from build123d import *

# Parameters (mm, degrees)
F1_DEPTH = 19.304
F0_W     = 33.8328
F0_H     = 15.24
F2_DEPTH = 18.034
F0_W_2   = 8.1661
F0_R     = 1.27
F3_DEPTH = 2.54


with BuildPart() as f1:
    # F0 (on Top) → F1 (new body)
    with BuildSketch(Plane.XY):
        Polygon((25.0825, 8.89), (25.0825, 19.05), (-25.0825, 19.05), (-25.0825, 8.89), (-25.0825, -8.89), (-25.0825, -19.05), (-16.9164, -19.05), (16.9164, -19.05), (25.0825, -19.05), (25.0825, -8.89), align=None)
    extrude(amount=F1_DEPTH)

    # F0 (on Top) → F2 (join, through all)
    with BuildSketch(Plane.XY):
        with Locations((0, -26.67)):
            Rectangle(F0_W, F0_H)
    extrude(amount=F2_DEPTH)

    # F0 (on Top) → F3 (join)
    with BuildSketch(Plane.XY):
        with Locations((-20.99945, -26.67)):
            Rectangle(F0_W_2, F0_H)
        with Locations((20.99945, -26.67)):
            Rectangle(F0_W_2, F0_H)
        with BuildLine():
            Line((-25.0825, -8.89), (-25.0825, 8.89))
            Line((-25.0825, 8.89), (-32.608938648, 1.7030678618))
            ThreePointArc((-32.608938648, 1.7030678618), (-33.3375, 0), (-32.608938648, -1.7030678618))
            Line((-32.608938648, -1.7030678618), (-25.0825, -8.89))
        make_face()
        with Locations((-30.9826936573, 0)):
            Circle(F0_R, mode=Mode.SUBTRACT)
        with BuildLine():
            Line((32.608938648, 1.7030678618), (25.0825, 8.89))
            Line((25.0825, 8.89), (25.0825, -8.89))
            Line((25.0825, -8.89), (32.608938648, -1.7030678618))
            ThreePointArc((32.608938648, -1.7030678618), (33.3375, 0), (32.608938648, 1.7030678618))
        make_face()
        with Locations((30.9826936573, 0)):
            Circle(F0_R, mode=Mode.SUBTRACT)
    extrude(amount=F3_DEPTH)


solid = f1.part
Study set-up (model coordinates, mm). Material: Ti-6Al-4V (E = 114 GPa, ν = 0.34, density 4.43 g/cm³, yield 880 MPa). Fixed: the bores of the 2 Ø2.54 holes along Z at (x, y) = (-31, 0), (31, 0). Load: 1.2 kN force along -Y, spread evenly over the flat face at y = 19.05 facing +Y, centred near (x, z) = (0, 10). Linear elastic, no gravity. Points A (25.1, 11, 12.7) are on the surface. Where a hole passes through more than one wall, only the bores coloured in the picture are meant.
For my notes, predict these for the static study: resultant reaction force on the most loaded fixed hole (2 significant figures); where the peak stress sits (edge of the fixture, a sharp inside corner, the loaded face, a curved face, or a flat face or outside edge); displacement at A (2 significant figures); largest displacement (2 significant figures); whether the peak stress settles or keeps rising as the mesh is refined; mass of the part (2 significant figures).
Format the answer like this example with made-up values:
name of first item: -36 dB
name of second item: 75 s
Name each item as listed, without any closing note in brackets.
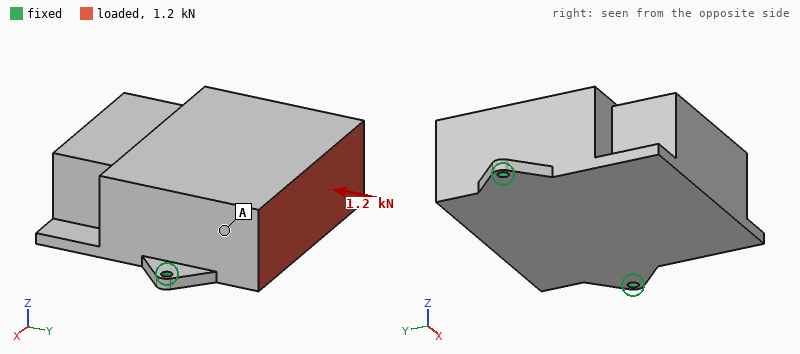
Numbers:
resultant reaction force on the most loaded fixed hole: 600 N
where the peak stress sits: edge of the fixture
displacement at A: 0.18 mm
largest displacement: 0.42 mm
whether the peak stress settles or keeps rising as the mesh is refined: keeps rising
mass of the part: 210 g
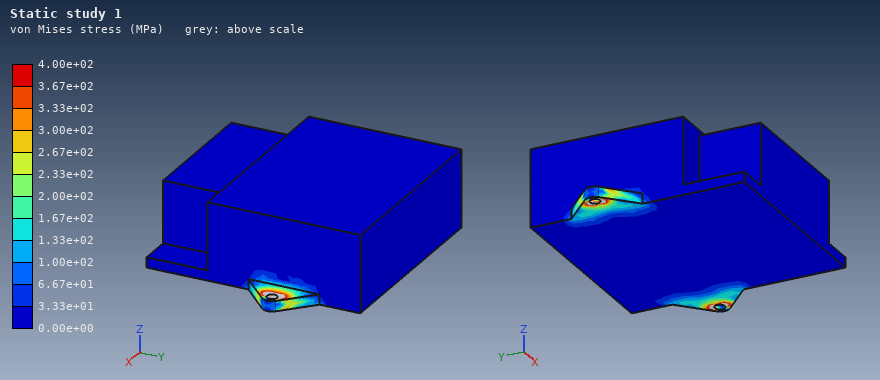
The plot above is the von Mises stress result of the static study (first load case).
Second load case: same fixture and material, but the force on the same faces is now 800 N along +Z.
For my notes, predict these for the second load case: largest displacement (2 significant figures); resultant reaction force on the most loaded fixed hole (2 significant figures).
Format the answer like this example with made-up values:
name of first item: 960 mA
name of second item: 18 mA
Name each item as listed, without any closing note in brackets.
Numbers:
largest displacement: 0.62 mm
resultant reaction force on the most loaded fixed hole: 460 N
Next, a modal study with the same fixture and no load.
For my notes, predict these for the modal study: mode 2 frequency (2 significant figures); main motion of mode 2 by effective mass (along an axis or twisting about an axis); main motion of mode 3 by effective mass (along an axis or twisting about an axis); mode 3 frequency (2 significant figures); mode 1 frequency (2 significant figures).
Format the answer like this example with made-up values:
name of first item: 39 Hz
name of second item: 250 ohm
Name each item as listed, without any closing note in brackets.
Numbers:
mode 2 frequency: 3300 Hz
main motion of mode 2 by effective mass: along Z
main motion of mode 3 by effective mass: along X
mode 3 frequency: 5100 Hz
mode 1 frequency: 570 Hz
